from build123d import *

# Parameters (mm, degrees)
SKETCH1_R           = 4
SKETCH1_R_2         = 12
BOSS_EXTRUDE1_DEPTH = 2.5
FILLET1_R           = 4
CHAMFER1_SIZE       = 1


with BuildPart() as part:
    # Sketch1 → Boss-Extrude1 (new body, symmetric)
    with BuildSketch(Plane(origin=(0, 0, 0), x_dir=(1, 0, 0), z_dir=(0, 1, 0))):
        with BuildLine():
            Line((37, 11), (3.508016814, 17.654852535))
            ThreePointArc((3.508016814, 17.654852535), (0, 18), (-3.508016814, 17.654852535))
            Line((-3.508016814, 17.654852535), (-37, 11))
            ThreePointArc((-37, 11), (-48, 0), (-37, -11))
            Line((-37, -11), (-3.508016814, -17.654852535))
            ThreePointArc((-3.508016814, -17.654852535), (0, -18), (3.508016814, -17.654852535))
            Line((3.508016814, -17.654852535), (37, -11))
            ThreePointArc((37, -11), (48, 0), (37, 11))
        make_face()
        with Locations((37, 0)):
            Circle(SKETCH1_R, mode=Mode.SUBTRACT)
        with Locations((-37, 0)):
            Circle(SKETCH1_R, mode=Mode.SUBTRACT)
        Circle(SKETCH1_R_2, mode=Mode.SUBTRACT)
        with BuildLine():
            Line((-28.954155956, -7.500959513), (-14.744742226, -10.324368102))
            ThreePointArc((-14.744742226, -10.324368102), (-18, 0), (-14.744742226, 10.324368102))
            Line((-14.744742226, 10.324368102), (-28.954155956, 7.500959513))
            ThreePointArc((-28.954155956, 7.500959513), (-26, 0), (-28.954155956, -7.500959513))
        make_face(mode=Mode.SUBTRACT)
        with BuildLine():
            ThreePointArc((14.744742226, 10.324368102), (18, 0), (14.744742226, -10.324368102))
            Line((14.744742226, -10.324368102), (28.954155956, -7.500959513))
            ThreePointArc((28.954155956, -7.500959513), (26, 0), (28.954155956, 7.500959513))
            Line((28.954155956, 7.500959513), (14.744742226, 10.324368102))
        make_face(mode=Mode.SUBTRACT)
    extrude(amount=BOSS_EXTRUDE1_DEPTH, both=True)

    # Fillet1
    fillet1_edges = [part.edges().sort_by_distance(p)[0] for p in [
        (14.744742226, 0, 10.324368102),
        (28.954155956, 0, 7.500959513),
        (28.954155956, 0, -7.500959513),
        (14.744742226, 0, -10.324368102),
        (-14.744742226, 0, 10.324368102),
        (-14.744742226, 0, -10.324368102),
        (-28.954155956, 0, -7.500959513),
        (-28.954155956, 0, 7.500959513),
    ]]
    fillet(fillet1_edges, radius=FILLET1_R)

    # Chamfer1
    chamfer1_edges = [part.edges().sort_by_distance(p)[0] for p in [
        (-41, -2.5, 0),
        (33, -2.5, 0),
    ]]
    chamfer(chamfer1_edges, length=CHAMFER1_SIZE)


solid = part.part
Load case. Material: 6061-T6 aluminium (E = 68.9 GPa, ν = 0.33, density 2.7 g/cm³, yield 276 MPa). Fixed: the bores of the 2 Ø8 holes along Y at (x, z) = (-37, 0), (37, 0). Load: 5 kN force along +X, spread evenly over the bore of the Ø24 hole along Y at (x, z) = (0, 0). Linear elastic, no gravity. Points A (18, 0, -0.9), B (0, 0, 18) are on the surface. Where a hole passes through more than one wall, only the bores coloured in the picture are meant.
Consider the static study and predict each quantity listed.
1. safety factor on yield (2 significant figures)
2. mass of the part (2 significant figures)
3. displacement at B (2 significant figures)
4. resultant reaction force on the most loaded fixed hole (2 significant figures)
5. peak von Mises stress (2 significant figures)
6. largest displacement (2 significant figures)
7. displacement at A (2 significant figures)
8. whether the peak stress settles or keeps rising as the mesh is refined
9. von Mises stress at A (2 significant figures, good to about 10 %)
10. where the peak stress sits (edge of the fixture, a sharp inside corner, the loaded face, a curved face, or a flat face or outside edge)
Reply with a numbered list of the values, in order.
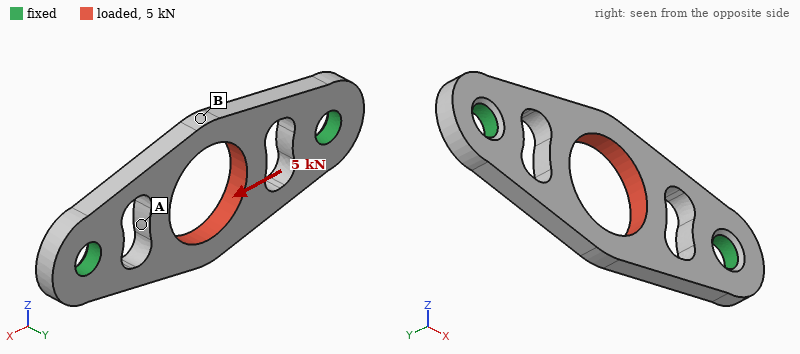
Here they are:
1. 2.1
2. 23 g
3. 20 µm
4. 2.5 kN
5. 130 MPa
6. 28 µm
7. 27 µm
8. settles
9. 44 MPa
10. a curved face
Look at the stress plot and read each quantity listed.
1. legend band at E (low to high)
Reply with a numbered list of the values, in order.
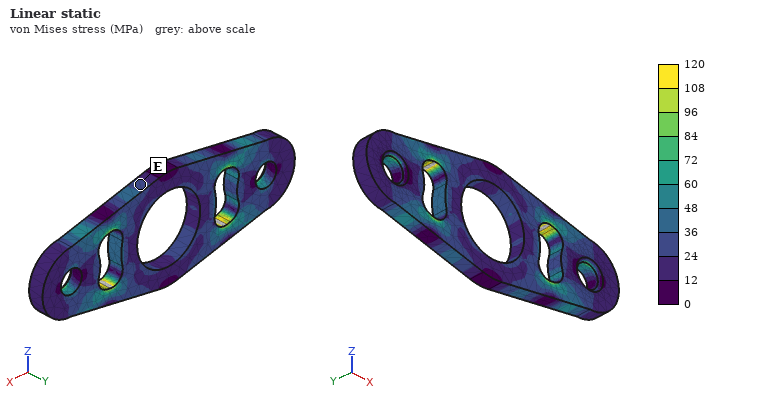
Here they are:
1. 24 to 36 MPa
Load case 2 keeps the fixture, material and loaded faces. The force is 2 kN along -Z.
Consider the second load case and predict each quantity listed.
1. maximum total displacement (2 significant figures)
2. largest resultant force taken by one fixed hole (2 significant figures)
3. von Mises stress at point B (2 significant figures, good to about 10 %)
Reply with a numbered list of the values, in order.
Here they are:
1. 44 µm
2. 1.0 kN
3. 31 MPa
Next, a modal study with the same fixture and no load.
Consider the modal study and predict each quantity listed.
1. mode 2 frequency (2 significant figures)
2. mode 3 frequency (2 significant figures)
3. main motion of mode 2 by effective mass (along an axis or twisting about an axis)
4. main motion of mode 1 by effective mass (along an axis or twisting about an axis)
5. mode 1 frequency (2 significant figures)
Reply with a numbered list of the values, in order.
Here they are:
1. 5200 Hz
2. 10 kHz
3. twisting about X
4. along Y
5. 4300 Hz
